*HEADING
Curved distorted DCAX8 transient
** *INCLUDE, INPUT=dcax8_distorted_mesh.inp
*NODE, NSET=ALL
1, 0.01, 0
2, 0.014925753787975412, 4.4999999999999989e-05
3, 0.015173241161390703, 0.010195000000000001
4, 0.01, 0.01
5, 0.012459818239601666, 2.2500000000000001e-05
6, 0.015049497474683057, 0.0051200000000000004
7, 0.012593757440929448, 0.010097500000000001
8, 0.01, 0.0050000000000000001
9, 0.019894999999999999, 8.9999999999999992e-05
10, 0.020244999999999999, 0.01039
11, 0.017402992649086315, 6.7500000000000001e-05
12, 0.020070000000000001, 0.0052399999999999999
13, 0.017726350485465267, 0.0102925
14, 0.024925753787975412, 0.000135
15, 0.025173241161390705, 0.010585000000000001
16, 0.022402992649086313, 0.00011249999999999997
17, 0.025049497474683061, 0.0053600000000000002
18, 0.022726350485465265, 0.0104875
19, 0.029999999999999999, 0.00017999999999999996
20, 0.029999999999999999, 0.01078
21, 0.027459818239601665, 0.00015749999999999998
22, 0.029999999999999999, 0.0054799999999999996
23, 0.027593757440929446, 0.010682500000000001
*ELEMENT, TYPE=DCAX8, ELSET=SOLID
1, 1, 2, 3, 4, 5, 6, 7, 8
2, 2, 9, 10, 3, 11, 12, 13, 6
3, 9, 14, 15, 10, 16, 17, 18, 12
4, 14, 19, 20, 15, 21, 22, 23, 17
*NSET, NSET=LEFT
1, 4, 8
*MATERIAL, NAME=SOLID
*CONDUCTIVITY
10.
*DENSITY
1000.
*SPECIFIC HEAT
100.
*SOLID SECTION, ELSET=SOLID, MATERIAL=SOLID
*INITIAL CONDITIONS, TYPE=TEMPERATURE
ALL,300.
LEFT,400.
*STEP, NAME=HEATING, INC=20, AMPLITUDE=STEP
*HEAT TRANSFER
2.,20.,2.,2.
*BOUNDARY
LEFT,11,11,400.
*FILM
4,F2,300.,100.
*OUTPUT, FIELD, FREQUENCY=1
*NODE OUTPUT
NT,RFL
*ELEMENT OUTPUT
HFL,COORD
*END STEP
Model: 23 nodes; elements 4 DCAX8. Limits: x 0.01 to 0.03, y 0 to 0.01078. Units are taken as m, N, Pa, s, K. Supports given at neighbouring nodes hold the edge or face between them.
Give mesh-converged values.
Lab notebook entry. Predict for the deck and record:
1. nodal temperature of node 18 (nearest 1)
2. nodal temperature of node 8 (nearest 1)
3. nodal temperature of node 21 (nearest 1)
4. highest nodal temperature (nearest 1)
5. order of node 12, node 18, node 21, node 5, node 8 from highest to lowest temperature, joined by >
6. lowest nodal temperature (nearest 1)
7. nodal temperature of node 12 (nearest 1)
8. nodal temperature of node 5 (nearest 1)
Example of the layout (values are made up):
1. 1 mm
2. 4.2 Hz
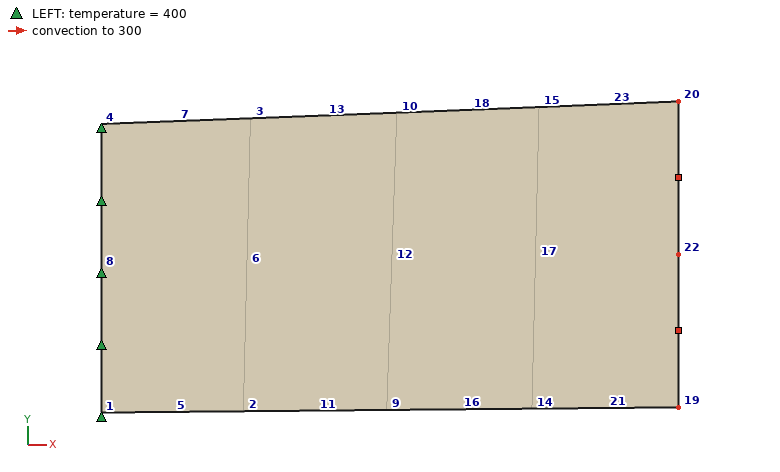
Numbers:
1. 381 K
2. 400 K
3. 377 K
4. 400 K
5. node 8 > node 5 > node 12 > node 18 > node 21
6. 374 K
7. 384 K
8. 395 K
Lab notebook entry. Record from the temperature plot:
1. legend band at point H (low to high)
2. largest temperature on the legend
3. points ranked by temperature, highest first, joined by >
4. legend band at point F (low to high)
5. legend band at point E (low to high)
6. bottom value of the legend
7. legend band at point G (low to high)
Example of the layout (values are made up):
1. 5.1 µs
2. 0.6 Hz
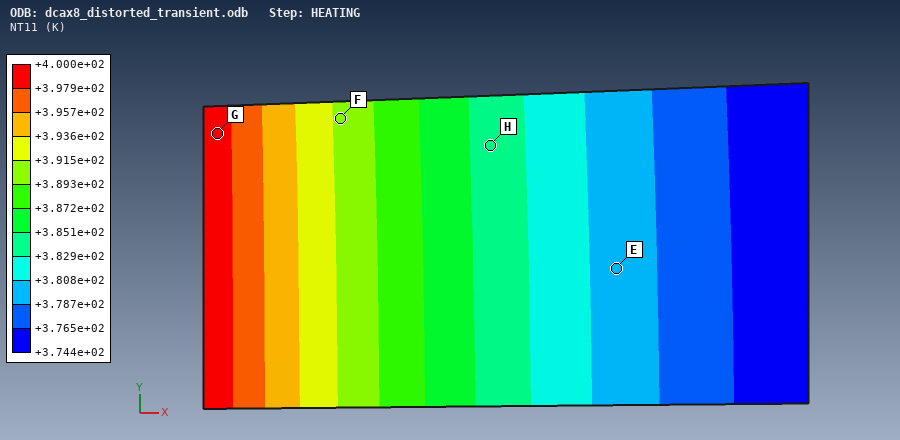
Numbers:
1. +3.829e+02 to +3.851e+02 K
2. +4.000e+02 K
3. G > F > H > E
4. +3.893e+02 to +3.915e+02 K
5. +3.787e+02 to +3.808e+02 K
6. +3.744e+02 K
7. +3.979e+02 to +4.000e+02 K
